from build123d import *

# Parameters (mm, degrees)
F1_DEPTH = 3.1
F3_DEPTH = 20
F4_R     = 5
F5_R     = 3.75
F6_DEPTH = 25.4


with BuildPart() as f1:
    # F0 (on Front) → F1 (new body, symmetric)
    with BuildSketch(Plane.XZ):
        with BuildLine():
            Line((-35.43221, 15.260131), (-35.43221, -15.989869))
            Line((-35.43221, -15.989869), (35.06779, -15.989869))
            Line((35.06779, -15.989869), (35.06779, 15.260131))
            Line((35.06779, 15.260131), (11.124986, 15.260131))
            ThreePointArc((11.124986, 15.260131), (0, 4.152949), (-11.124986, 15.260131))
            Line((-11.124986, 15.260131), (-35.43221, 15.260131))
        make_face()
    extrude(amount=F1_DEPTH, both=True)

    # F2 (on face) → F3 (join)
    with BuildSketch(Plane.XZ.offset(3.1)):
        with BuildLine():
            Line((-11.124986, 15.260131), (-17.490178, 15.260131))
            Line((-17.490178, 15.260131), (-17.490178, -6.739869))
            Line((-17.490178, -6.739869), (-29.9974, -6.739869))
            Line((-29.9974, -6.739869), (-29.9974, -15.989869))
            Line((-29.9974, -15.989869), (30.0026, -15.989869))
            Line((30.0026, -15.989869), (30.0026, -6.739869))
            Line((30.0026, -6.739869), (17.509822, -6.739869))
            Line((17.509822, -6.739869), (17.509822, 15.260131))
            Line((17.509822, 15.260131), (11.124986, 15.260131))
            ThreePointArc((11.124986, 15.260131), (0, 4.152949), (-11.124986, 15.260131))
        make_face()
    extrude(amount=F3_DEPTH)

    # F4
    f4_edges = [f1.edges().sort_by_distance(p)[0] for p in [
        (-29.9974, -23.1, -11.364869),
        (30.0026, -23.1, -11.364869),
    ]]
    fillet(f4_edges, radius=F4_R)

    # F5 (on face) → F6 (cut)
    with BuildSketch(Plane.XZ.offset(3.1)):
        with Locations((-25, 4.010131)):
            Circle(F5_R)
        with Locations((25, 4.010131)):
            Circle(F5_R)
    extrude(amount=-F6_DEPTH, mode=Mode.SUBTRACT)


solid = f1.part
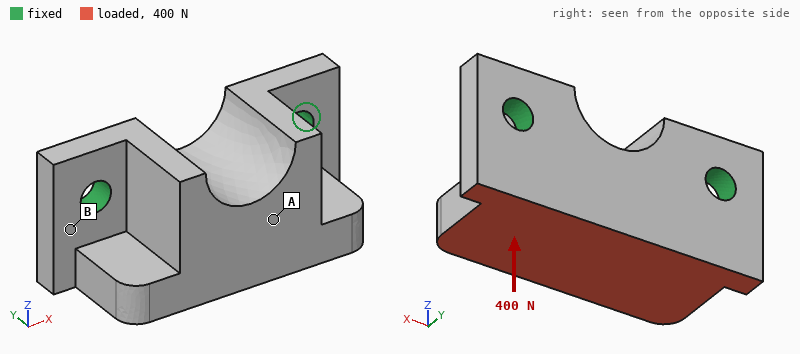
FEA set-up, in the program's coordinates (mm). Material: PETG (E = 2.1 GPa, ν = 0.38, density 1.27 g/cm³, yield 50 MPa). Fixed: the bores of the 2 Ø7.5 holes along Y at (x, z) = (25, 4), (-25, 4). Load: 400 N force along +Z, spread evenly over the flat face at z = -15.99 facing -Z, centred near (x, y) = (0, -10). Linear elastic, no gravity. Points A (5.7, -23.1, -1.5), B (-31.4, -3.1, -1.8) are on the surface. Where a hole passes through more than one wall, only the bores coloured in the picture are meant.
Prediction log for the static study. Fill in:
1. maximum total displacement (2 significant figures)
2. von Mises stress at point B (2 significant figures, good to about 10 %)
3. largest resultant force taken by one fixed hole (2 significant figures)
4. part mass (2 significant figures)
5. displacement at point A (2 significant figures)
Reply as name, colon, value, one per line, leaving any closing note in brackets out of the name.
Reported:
maximum total displacement: 0.22 mm
von Mises stress at point B: 4.2 MPa
largest resultant force taken by one fixed hole: 210 N
part mass: 44 g
displacement at point A: 0.17 mm
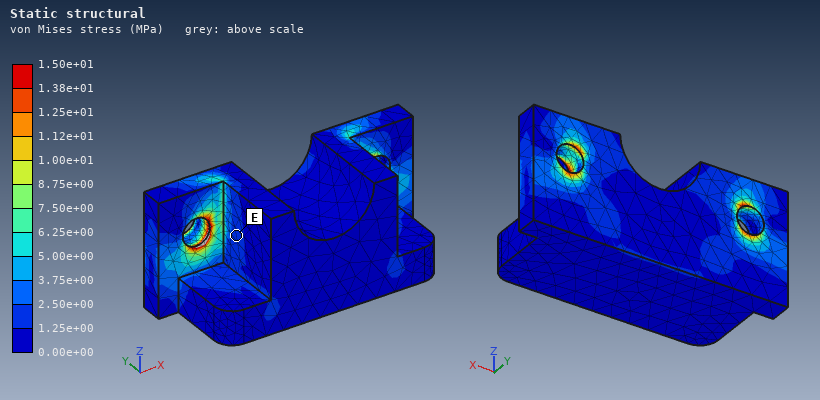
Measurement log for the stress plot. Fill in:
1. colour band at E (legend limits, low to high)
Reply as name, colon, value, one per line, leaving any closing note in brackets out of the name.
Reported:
colour band at E: 1.25e+00 to 2.50e+00 MPa
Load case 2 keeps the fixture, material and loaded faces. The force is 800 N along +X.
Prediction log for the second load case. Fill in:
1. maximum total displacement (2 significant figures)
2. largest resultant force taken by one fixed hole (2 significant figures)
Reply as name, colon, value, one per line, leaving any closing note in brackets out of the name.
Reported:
maximum total displacement: 90 µm
largest resultant force taken by one fixed hole: 520 N
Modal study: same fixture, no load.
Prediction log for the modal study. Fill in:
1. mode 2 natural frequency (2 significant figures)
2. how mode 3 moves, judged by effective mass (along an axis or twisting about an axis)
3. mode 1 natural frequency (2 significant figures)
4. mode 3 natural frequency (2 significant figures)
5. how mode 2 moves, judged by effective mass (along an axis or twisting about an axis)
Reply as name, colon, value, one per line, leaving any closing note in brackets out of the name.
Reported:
mode 2 natural frequency: 3100 Hz
how mode 3 moves, judged by effective mass: along Y
mode 1 natural frequency: 1200 Hz
mode 3 natural frequency: 3200 Hz
how mode 2 moves, judged by effective mass: along X
